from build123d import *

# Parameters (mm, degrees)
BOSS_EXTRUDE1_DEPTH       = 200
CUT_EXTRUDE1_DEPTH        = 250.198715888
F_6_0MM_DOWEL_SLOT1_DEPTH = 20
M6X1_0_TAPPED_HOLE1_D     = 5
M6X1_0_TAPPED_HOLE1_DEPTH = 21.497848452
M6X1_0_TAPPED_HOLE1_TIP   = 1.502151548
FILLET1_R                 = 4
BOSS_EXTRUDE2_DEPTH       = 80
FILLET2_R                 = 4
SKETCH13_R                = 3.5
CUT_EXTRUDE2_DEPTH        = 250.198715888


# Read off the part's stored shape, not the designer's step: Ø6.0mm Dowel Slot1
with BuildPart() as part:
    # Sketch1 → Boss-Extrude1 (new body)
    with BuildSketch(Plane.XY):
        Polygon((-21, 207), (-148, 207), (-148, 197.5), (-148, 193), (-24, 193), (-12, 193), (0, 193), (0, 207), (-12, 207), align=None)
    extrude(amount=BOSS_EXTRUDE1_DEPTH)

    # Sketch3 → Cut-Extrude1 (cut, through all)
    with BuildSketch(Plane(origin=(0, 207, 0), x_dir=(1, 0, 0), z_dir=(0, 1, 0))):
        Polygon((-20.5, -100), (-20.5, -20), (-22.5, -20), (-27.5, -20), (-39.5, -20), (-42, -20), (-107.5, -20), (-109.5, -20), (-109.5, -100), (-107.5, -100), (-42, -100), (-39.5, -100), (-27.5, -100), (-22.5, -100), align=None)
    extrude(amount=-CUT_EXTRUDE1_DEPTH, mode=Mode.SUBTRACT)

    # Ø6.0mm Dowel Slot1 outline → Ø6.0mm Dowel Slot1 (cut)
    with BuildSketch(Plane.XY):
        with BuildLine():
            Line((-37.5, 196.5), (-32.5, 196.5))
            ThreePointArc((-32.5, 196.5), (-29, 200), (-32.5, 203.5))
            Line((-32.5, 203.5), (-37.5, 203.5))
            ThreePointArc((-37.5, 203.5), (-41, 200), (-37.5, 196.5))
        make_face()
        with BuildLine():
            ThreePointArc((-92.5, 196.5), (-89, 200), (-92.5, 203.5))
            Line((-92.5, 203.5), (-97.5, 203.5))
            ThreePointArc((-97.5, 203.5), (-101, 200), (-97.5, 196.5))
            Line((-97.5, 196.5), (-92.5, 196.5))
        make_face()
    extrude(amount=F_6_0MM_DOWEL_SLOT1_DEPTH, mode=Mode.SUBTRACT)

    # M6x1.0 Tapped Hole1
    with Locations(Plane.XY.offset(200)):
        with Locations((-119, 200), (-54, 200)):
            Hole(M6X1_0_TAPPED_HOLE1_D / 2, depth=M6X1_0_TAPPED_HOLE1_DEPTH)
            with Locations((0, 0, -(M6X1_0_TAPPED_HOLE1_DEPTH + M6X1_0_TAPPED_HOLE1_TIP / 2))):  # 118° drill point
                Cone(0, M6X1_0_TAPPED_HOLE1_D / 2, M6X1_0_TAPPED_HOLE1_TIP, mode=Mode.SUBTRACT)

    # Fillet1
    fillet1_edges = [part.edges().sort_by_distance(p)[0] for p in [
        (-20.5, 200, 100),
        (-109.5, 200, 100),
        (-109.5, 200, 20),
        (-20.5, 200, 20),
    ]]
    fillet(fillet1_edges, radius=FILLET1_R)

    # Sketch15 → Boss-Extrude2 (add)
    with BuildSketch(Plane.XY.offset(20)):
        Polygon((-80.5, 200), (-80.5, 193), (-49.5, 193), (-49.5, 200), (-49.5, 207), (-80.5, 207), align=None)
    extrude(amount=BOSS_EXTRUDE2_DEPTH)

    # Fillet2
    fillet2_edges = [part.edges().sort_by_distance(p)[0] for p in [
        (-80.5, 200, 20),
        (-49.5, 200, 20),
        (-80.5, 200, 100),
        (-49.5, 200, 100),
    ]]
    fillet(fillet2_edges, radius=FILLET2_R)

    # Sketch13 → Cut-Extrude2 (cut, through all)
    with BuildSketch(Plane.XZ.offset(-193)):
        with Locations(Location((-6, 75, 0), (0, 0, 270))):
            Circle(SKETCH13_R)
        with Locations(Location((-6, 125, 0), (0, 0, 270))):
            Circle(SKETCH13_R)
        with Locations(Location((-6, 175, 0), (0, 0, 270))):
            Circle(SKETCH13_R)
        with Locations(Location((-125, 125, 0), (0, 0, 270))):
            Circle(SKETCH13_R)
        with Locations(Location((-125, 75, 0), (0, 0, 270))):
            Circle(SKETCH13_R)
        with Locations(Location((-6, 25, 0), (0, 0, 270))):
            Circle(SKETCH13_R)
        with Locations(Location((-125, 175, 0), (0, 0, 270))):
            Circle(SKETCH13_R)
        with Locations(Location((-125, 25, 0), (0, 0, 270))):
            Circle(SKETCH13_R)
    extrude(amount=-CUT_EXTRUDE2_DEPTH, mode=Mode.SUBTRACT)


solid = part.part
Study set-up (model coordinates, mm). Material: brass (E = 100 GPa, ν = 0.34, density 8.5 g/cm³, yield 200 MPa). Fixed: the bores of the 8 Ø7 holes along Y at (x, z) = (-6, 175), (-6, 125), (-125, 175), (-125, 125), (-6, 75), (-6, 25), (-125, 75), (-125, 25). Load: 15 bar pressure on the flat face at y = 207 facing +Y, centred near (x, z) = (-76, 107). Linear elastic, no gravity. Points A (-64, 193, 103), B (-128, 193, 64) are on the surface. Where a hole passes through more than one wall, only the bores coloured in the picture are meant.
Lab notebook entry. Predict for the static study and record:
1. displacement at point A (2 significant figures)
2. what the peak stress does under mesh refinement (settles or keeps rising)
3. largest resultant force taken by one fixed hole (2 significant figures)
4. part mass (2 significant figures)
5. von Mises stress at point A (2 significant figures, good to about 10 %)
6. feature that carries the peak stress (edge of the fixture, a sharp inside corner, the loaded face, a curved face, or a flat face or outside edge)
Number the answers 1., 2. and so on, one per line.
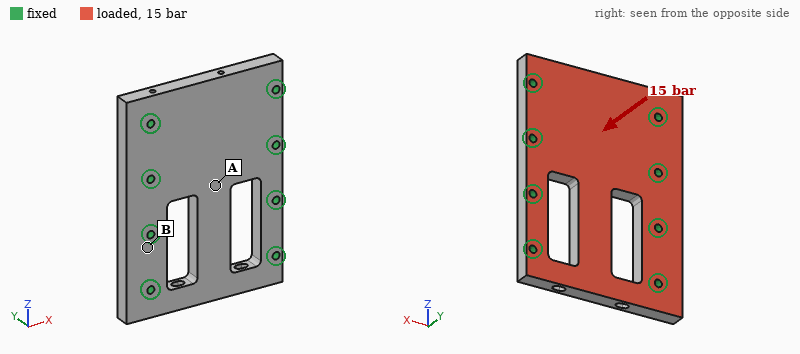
1. 0.077 mm
2. keeps rising
3. 6.7 kN
4. 2.9 kg
5. 40 MPa
6. edge of the fixture
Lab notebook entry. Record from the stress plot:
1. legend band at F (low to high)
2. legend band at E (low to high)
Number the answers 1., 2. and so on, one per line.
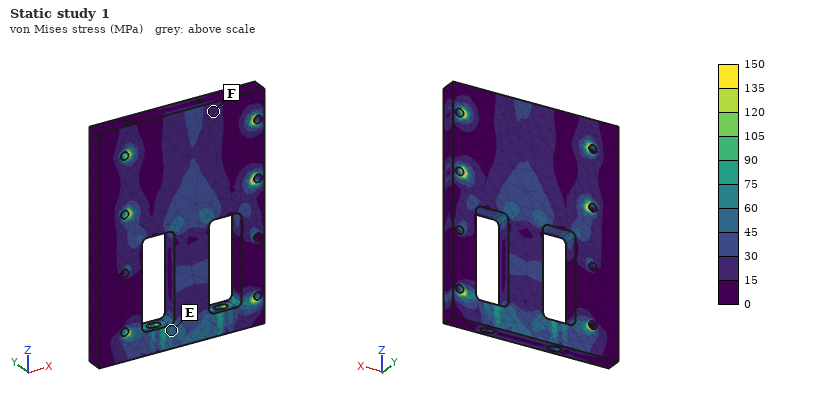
1. 15 to 30 MPa
2. 45 to 60 MPa
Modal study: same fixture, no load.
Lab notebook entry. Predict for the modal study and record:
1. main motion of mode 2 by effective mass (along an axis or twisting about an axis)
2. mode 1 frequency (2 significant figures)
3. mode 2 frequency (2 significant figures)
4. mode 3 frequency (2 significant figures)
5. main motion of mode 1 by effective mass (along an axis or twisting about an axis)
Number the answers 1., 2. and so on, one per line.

1. along Y
2. 1900 Hz
3. 2800 Hz
4. 3200 Hz
5. along Y
